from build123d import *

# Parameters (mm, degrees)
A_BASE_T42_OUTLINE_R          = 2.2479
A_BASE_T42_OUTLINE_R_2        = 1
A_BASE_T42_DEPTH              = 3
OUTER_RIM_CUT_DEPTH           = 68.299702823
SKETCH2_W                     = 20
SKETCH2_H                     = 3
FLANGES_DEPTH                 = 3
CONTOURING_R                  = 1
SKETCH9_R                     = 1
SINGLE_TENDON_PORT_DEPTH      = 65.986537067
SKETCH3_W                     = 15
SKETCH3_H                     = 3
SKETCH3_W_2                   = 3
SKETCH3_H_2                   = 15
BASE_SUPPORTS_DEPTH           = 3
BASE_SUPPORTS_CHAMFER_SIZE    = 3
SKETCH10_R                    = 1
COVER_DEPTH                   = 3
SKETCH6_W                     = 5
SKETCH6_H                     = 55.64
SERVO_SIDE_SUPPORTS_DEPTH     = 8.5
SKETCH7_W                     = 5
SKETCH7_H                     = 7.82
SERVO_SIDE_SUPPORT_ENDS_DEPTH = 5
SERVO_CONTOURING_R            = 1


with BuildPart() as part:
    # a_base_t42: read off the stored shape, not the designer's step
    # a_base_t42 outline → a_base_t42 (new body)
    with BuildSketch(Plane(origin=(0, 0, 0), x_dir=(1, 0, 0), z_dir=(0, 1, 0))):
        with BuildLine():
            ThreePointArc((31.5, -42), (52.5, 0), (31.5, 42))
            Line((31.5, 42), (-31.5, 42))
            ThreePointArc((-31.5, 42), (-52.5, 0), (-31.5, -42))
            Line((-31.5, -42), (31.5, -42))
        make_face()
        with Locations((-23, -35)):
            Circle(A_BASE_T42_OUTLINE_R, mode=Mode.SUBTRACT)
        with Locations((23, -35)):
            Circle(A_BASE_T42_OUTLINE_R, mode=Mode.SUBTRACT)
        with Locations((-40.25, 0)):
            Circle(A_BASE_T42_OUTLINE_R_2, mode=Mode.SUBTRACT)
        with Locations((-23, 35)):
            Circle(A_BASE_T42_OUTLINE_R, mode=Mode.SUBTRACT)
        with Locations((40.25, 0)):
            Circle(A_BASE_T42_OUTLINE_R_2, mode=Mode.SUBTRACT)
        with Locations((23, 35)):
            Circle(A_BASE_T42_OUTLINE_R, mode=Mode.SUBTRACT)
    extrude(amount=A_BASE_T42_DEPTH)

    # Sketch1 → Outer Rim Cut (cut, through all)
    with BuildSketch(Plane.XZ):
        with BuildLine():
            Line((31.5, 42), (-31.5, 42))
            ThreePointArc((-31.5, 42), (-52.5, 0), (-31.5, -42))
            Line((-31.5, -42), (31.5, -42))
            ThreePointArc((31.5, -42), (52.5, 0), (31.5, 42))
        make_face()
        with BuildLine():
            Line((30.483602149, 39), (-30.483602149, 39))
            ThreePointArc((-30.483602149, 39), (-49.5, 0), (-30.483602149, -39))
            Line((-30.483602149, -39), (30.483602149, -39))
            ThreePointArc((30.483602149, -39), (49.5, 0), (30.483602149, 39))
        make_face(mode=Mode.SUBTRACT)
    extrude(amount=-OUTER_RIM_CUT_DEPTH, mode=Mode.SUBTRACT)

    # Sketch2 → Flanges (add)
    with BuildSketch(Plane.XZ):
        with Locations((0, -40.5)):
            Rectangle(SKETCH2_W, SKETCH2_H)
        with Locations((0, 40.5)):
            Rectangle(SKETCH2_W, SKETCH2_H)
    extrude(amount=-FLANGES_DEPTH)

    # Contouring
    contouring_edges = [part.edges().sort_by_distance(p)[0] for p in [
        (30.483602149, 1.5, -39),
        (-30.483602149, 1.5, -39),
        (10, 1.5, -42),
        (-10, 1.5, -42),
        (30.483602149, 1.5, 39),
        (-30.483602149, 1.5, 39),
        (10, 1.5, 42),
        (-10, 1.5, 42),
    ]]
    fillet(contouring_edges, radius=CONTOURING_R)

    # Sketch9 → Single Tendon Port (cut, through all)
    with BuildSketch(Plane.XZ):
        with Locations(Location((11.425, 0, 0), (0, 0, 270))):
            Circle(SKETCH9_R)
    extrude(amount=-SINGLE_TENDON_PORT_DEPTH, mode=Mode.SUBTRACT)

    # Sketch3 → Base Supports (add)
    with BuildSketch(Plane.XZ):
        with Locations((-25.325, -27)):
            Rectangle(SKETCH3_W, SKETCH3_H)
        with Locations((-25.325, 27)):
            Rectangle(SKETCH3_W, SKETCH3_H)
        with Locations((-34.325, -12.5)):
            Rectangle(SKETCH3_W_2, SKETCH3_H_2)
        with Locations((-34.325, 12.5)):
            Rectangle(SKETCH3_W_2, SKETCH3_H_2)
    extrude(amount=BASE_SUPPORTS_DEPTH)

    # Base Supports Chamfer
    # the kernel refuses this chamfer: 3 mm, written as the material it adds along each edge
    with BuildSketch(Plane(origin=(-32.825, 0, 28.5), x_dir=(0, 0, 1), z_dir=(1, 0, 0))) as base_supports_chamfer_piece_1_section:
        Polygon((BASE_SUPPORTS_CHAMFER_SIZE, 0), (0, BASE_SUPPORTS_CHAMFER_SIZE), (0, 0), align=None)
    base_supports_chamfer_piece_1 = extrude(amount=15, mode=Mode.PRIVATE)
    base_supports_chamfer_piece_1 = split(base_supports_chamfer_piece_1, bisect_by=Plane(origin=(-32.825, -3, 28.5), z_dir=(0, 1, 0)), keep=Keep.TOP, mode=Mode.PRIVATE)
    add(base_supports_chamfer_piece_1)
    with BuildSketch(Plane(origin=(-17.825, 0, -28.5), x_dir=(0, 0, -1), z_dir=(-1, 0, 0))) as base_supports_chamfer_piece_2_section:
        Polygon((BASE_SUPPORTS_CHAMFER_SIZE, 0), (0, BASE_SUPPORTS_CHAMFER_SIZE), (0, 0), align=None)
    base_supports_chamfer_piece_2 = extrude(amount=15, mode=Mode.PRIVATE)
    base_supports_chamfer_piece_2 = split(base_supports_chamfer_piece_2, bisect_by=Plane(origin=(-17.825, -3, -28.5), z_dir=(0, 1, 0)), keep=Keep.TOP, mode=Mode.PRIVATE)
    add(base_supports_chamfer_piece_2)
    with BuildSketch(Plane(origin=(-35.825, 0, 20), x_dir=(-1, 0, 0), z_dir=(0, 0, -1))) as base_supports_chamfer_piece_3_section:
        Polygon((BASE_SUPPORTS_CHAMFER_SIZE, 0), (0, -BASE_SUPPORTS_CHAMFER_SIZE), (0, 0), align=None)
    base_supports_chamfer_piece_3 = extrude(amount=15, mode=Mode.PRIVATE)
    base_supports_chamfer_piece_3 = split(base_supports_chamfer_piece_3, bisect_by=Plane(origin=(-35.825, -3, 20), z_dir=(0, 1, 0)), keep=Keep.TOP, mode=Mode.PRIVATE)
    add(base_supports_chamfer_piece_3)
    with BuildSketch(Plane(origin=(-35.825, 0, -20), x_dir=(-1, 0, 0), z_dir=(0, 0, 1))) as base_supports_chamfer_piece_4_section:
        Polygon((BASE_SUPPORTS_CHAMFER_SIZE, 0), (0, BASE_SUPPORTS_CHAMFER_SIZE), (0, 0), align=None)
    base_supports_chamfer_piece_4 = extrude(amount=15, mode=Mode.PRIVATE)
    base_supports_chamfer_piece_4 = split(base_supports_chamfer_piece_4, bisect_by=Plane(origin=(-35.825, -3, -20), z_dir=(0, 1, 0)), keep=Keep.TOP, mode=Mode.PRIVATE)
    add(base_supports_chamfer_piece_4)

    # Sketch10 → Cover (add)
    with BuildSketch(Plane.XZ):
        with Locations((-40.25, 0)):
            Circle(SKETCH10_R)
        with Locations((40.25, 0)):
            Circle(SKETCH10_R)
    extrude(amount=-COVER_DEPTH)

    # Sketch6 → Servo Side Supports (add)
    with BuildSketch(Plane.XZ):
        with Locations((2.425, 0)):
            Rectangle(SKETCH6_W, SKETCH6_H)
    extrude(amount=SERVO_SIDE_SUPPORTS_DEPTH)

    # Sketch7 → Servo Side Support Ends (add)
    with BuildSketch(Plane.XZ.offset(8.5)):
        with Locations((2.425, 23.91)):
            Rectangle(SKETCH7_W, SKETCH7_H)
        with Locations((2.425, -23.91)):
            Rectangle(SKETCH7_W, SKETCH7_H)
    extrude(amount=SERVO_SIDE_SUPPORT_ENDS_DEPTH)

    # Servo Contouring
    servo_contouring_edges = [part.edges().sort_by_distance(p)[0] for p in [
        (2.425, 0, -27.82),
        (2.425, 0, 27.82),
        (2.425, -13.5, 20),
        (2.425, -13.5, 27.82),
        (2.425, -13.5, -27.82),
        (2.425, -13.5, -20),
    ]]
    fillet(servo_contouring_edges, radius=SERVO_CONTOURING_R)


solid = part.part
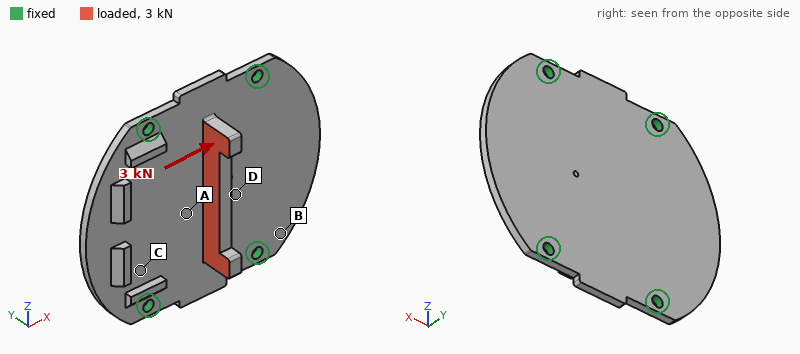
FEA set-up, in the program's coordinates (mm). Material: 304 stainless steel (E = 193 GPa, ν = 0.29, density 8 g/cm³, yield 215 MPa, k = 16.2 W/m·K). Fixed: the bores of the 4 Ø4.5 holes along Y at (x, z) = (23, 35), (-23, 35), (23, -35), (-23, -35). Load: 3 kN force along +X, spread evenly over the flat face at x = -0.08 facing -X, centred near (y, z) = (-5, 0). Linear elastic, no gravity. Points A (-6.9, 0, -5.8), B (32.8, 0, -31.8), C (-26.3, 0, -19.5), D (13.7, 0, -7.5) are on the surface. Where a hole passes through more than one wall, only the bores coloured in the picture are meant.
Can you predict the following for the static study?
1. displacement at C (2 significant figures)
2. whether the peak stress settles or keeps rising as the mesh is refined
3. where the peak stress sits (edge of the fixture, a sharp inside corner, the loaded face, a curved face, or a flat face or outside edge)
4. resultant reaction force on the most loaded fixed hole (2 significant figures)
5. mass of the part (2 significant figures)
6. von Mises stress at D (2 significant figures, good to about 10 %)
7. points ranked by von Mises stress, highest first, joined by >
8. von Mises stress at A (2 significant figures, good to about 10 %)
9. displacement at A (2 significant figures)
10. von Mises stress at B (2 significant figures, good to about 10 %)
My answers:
9.5 µm
keeps rising
a sharp inside corner
840 N
190 g
44 MPa
A > D > B > C
57 MPa
20 µm
20 MPa
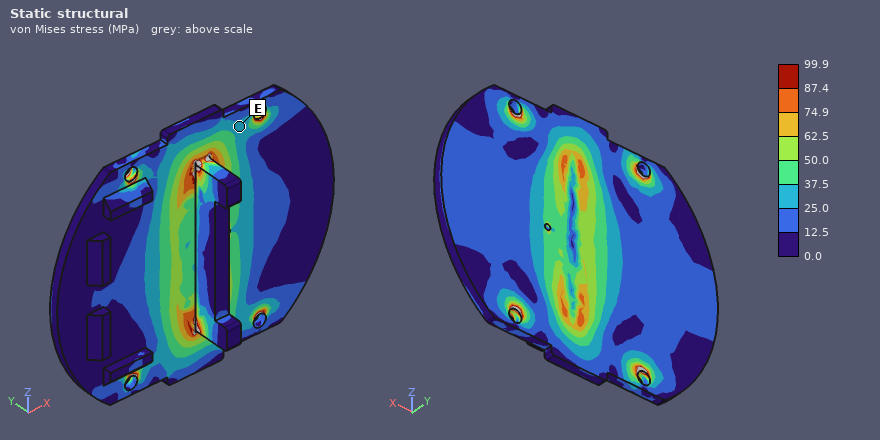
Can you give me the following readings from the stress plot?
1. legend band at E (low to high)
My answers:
25.0 to 37.5 MPa
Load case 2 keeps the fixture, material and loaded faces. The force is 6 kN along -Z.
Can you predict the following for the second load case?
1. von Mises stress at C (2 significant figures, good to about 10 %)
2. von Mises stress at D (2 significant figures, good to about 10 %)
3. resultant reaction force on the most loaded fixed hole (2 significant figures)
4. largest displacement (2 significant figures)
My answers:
19 MPa
38 MPa
1.7 kN
41 µm
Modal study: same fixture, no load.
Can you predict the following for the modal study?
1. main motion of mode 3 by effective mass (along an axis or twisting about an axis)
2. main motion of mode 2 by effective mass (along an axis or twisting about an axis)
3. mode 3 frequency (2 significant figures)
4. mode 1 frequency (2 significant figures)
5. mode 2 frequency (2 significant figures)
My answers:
along Y
along Y
3500 Hz
2400 Hz
2600 Hz
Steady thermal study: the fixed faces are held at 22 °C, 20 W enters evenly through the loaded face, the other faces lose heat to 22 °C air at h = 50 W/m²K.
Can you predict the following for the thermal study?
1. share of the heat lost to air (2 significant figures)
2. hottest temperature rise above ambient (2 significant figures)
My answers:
73 %
77 K
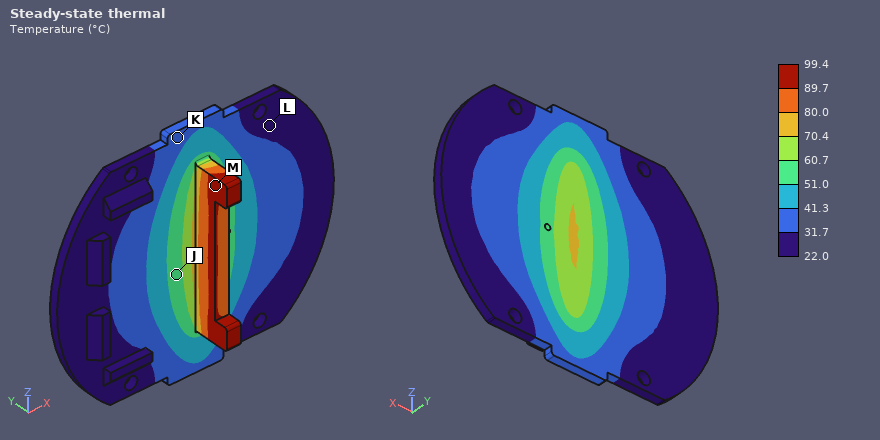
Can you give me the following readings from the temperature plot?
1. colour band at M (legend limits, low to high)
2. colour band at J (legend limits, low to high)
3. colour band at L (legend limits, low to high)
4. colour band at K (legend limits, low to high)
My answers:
89.7 to 99.4 °C
51.0 to 60.7 °C
22.0 to 31.7 °C
31.7 to 41.3 °C
